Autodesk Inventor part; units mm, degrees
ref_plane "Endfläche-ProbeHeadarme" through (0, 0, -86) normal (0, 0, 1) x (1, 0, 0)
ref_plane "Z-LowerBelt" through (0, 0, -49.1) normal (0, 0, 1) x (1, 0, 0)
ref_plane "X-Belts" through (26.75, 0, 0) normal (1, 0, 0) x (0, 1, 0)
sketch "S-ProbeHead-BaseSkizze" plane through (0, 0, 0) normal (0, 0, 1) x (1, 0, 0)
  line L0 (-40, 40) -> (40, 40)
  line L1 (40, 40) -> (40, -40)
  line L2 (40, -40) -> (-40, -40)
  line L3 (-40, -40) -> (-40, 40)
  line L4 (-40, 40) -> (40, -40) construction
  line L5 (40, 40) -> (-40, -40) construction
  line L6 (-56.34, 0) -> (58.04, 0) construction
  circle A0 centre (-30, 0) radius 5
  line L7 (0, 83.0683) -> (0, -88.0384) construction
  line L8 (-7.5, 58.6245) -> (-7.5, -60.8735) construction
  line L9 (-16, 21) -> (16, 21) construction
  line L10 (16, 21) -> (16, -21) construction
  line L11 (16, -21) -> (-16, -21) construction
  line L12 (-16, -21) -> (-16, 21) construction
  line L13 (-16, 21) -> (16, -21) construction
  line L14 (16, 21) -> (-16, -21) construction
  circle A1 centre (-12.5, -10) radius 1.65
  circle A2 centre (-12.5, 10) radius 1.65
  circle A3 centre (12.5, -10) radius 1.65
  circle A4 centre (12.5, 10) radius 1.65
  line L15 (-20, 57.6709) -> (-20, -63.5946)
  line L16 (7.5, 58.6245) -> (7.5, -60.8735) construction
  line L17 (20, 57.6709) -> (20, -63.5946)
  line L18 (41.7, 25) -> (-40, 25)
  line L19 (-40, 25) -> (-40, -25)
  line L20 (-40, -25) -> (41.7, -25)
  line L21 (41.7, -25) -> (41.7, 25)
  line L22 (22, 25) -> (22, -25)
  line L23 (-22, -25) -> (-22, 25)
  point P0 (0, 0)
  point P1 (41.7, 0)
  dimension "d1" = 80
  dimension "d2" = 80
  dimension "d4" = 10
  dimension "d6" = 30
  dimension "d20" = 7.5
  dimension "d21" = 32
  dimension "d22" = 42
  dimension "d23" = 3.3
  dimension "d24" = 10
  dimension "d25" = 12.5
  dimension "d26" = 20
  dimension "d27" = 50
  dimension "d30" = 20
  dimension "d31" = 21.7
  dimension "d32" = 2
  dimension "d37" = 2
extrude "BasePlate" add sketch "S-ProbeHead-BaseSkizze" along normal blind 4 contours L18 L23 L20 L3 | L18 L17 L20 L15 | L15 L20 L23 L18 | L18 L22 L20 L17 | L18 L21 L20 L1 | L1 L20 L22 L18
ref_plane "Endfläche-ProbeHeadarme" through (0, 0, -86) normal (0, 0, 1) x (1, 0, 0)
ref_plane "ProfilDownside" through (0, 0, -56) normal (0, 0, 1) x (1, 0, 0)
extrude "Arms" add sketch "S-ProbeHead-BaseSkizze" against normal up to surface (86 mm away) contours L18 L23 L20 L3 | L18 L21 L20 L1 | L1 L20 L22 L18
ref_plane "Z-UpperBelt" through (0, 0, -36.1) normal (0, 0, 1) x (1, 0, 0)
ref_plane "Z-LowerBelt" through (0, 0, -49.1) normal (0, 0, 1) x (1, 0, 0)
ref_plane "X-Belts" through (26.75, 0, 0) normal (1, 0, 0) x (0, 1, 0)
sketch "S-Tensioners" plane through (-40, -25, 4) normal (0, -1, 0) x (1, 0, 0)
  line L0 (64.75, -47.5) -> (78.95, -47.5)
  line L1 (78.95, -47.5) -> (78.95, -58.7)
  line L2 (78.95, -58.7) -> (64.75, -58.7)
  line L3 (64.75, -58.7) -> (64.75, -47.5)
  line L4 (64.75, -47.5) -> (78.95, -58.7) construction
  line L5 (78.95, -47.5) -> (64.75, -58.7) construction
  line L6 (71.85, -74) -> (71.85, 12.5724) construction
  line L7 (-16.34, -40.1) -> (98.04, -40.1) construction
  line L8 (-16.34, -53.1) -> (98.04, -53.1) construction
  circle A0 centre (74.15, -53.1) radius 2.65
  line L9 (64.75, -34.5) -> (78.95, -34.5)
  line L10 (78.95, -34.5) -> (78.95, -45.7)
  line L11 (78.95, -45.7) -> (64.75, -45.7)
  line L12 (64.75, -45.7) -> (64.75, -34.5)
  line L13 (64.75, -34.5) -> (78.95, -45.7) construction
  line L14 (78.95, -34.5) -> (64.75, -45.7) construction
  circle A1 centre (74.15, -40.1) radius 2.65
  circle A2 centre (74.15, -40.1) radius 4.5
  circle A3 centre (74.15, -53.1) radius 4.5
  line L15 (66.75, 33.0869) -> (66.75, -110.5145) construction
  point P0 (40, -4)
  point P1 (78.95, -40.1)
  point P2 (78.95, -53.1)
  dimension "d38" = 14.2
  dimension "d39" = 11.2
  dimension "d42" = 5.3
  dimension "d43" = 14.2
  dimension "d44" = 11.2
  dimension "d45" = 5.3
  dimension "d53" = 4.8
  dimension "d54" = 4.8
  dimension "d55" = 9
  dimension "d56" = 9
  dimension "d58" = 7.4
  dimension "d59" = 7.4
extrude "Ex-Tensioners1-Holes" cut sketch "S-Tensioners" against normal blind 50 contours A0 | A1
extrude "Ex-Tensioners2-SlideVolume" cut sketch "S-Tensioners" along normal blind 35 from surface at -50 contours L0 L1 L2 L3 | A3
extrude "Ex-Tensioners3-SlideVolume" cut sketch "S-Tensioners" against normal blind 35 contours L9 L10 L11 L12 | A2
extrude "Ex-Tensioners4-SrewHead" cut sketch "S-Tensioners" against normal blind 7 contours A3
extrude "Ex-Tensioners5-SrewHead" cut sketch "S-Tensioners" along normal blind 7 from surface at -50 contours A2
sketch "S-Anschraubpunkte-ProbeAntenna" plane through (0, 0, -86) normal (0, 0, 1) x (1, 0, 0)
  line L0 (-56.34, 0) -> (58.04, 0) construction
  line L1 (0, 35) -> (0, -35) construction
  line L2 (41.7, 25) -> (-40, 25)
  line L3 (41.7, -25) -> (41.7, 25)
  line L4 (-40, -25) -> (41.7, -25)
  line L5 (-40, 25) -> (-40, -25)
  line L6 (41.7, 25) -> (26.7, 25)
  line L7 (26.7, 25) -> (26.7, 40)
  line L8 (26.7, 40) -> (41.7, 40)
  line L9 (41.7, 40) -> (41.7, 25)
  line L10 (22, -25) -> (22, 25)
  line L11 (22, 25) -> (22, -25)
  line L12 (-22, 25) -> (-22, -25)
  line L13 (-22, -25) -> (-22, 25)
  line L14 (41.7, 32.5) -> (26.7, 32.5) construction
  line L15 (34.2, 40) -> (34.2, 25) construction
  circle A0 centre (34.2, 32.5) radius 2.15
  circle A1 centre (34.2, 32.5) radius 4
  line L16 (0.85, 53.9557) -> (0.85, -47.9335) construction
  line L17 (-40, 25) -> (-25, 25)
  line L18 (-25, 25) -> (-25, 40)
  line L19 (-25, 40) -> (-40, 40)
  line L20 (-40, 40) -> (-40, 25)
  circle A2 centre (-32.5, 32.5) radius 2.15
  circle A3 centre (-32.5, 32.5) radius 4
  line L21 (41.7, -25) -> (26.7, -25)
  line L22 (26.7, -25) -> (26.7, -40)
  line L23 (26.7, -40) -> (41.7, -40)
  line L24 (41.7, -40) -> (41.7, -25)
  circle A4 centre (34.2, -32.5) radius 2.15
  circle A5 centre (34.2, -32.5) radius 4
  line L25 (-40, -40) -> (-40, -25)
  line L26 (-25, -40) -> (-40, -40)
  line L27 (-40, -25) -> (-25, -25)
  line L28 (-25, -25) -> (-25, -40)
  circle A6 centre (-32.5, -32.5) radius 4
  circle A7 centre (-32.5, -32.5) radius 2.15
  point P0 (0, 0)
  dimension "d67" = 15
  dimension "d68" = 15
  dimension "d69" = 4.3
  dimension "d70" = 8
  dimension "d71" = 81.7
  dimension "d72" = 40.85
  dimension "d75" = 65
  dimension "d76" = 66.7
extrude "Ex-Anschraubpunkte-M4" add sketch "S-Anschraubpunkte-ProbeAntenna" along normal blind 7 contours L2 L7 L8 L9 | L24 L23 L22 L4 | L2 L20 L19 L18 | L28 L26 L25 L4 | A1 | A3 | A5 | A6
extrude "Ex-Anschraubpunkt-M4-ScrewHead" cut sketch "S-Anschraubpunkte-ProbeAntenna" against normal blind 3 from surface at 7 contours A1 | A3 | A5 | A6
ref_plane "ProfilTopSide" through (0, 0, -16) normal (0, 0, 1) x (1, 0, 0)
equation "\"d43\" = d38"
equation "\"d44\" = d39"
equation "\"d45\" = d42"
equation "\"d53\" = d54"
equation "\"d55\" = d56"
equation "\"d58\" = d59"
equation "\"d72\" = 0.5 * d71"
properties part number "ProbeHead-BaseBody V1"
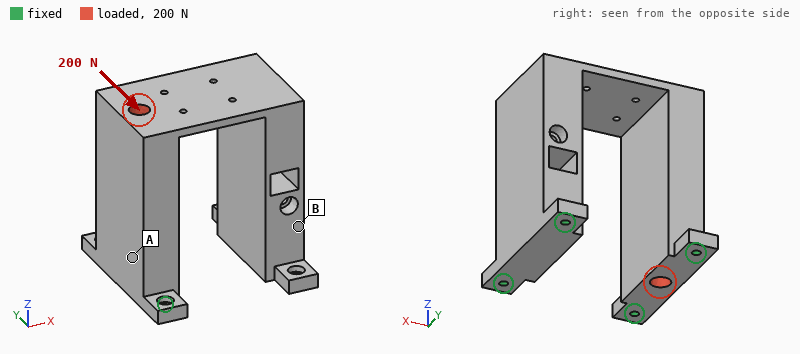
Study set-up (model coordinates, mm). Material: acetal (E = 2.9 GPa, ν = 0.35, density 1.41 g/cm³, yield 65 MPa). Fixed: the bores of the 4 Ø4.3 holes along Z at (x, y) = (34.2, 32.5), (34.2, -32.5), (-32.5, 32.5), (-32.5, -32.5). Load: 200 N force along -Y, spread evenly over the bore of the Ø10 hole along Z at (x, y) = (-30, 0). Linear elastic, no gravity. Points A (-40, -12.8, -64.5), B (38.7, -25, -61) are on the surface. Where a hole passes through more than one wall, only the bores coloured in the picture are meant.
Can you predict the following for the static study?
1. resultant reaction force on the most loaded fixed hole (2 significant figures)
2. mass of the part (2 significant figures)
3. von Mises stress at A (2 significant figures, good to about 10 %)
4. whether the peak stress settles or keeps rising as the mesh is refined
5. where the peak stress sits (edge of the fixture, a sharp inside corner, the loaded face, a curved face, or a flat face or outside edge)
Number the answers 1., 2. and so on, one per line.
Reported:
1. 140 N
2. 230 g
3. 0.70 MPa
4. keeps rising
5. edge of the fixture
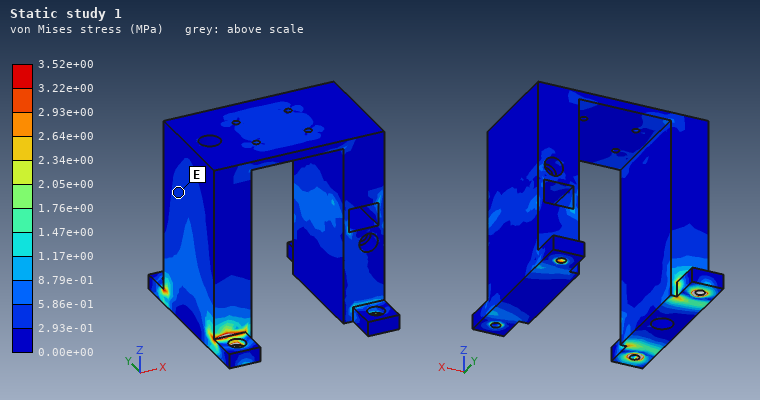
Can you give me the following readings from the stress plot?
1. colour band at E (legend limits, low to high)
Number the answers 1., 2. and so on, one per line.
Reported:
1. 2.93e-01 to 5.86e-01 MPa
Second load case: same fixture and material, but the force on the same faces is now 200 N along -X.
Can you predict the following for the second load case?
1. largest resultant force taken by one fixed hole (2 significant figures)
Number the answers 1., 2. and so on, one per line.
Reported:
1. 87 N
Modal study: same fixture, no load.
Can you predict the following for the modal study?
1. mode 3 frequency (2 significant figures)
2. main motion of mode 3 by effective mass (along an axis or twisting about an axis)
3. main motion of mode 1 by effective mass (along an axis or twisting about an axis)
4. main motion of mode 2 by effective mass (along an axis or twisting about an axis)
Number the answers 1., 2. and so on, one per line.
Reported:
1. 840 Hz
2. twisting about Z
3. along X
4. along Y
